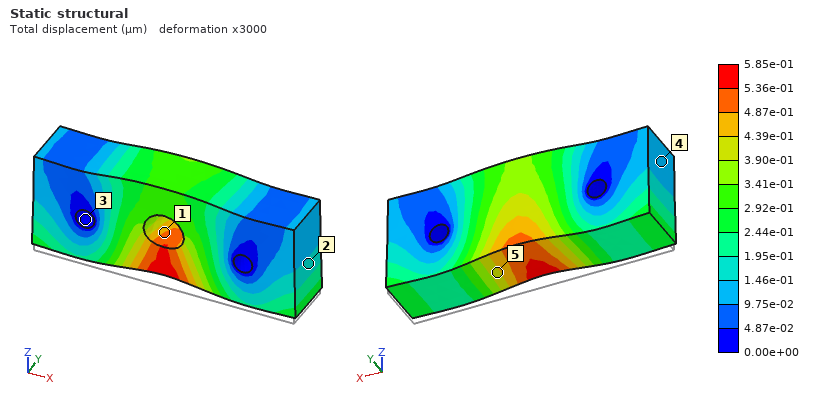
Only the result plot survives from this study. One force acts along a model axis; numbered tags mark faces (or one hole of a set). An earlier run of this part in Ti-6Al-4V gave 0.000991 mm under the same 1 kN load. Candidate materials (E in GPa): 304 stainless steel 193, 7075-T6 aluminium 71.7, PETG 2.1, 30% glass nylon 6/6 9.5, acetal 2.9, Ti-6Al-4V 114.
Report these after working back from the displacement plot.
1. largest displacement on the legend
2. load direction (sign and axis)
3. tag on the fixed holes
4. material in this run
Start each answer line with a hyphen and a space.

- 5.85e-01 µm
- +Z
- 3
- 304 stainless steel
